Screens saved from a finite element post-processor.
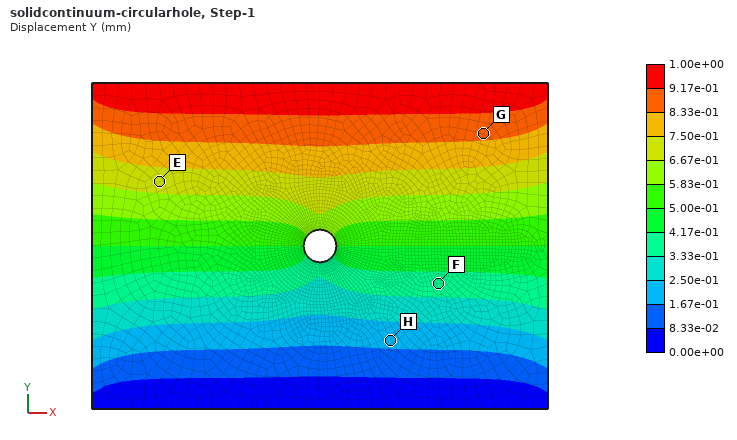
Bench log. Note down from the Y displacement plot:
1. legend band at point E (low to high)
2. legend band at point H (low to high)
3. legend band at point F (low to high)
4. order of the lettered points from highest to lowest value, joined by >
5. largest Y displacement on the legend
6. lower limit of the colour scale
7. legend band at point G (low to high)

6.67e-01 to 7.50e-01 mm
1.67e-01 to 2.50e-01 mm
3.33e-01 to 4.17e-01 mm
G > E > F > H
1.00e+00 mm
0.00e+00 mm
8.33e-01 to 9.17e-01 mm
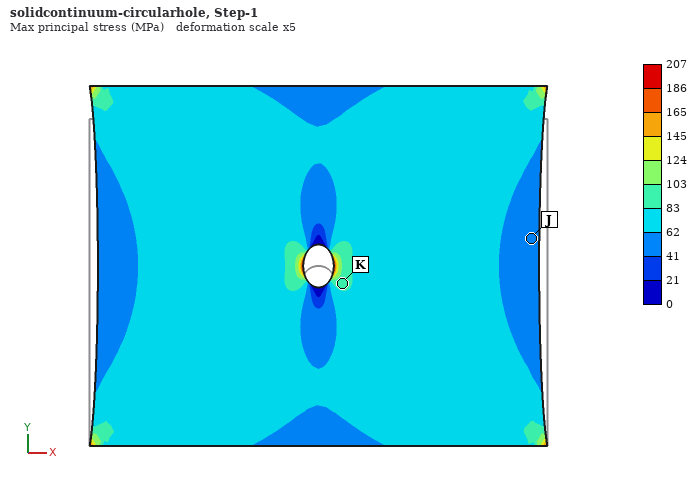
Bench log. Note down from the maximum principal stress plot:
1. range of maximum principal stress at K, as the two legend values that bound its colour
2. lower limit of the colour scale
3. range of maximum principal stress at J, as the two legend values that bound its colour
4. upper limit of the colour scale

83 to 103 MPa
0 MPa
41 to 62 MPa
207 MPa
